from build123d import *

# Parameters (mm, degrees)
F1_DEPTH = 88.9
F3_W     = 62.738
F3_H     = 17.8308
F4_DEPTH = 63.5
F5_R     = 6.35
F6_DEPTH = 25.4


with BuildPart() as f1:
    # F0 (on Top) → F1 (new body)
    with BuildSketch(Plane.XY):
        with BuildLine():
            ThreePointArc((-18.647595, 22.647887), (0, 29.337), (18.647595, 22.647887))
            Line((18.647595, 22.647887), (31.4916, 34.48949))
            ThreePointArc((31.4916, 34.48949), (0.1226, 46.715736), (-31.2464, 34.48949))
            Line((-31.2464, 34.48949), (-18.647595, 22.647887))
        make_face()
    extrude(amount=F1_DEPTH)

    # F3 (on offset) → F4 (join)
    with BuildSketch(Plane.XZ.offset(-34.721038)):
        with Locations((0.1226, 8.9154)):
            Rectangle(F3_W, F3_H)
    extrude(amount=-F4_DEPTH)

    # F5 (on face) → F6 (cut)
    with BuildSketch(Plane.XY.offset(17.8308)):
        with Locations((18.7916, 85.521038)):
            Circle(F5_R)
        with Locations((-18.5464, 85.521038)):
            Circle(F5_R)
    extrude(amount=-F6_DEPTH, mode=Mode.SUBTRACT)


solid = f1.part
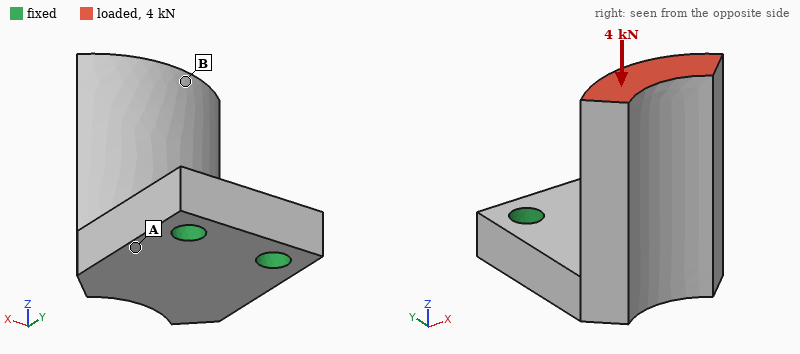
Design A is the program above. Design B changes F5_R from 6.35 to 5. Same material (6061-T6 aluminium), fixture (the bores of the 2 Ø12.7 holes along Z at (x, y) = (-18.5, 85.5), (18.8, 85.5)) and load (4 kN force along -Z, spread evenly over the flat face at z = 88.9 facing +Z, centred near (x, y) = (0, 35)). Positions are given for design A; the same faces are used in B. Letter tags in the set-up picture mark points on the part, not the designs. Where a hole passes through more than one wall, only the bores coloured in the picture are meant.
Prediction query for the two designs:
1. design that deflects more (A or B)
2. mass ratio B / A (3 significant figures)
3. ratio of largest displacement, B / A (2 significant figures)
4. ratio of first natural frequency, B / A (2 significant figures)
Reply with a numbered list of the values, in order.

1. B
2. 1.01
3. 1.1
4. 0.97
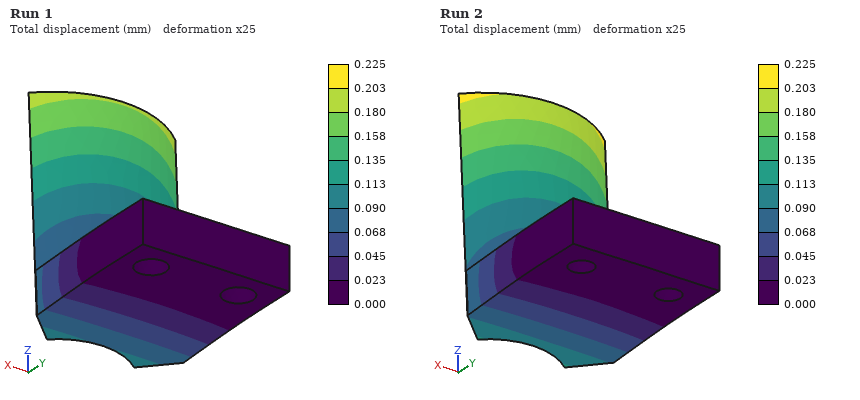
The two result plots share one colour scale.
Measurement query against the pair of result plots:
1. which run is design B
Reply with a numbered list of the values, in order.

1. Run 2
